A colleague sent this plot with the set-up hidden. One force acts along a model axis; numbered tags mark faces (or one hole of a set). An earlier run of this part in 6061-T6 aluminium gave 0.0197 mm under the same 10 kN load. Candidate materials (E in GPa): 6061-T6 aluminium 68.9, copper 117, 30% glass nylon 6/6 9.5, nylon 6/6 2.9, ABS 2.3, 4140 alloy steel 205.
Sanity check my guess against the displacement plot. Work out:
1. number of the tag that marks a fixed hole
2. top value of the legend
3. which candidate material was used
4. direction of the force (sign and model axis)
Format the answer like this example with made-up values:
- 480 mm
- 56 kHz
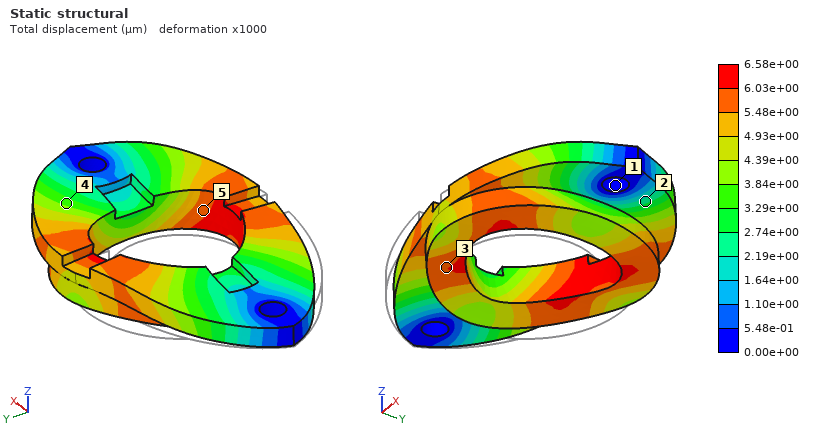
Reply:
- 1
- 6.58e+00 µm
- 4140 alloy steel
- +X
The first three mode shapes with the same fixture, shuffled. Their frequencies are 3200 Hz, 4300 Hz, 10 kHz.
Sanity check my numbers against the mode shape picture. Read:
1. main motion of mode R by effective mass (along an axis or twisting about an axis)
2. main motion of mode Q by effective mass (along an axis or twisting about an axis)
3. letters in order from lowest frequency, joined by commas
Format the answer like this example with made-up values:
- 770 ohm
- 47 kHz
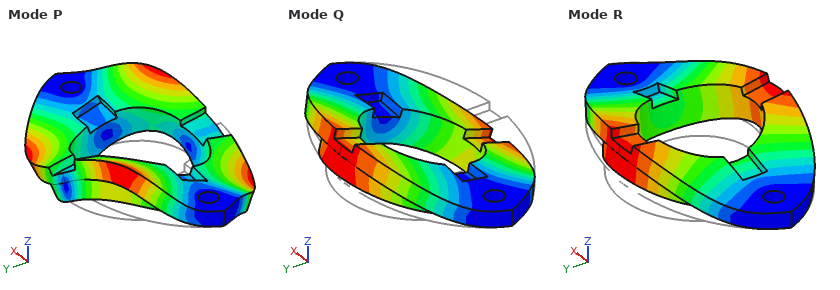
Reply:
- along Z
- twisting about X
- Q, R, P
